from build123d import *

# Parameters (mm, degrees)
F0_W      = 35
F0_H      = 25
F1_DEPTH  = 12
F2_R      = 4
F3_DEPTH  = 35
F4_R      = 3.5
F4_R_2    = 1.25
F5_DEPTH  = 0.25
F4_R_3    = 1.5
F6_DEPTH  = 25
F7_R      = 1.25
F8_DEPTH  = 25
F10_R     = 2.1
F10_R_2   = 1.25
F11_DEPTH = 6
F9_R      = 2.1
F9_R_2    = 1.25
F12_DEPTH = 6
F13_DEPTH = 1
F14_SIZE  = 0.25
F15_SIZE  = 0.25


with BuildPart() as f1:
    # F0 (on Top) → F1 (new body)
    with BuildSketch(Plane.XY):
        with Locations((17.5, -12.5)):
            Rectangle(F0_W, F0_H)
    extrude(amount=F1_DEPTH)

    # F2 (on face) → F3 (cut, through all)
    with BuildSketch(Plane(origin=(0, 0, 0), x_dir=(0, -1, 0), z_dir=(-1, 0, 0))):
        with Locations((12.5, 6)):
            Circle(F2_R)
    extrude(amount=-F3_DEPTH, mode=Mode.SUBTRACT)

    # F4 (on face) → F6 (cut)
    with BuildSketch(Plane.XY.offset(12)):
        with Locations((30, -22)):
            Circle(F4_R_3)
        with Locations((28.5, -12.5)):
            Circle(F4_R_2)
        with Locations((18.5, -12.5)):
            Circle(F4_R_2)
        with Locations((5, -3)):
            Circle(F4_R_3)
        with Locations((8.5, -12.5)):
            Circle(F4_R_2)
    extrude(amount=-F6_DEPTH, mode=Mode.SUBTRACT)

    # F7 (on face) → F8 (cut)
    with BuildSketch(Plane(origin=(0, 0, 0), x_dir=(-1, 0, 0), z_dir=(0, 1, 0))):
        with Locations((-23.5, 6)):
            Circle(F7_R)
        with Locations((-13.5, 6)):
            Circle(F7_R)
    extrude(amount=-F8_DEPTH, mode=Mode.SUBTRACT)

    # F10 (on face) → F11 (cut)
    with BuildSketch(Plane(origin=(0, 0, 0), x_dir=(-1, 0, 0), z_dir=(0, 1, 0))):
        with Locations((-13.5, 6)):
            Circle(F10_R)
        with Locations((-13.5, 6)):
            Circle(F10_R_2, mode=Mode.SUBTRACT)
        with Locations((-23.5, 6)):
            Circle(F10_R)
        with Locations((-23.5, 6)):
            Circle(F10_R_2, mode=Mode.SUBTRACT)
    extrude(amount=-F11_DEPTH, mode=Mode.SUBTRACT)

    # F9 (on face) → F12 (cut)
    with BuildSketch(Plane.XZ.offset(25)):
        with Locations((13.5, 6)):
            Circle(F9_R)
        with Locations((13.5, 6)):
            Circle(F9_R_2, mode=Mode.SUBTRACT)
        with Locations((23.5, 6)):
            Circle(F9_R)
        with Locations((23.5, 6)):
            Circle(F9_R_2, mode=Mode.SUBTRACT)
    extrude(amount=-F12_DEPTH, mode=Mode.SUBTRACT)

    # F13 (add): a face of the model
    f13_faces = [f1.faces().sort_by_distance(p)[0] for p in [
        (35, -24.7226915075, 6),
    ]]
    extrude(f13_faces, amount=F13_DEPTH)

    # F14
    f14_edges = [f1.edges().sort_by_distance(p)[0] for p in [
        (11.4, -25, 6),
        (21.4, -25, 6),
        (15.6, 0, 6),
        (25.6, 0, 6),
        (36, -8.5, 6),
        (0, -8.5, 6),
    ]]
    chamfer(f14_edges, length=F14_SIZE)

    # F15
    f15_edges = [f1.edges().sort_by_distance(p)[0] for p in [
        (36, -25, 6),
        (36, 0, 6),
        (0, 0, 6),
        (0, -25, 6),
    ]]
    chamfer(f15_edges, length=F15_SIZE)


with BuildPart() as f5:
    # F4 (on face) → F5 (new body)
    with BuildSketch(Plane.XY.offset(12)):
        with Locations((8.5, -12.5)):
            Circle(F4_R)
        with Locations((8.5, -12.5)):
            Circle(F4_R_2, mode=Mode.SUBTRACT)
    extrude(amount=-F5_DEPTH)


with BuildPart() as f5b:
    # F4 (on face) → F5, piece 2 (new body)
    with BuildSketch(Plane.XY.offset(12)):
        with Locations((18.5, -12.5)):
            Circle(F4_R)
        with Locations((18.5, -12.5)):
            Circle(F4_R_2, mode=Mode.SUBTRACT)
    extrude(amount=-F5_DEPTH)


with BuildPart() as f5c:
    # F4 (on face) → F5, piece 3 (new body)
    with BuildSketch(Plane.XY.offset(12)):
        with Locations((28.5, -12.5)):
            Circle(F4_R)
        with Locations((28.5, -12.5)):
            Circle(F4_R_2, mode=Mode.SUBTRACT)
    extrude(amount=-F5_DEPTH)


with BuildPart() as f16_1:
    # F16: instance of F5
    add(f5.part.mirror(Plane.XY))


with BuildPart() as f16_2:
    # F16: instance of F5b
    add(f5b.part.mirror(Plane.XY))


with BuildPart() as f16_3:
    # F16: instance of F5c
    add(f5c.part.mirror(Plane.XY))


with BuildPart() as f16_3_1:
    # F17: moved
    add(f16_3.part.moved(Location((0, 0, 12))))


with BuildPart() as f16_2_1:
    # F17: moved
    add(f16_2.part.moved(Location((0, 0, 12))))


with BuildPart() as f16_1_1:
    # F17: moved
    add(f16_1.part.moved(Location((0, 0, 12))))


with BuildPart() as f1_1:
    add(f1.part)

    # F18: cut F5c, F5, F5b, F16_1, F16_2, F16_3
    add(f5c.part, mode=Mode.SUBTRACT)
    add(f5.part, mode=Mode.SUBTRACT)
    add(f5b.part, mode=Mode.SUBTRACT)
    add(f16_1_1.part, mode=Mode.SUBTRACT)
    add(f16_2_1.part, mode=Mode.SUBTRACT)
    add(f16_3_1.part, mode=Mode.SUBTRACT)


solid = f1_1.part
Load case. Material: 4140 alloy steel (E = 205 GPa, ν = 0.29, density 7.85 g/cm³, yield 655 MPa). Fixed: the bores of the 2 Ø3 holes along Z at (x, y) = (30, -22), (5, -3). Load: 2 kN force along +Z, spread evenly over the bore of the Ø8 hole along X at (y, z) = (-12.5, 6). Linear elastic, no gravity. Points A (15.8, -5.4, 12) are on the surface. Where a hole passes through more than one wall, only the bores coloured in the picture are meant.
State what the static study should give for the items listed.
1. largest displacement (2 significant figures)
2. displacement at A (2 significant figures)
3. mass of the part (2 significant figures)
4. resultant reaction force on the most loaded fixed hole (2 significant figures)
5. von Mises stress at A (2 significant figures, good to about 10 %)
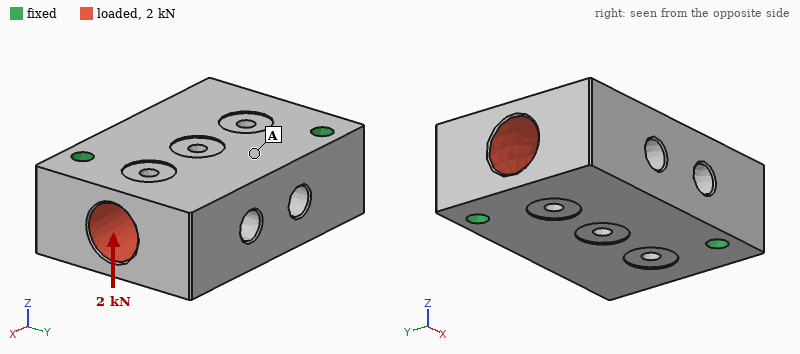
3.3 µm
1.6 µm
65 g
1.0 kN
5.9 MPa
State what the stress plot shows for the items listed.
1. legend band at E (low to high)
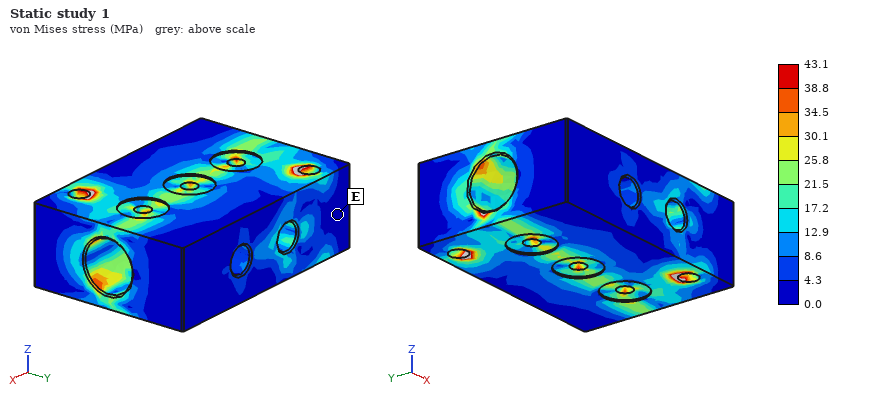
0.0 to 4.3 MPa
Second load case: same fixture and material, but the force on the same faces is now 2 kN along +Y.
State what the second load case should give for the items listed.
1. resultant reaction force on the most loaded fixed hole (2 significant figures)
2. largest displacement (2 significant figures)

1.0 kN
0.97 µm
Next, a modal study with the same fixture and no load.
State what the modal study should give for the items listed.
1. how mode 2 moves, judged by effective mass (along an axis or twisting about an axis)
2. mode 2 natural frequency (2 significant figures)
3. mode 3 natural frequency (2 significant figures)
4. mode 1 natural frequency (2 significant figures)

along Z
18 kHz
30 kHz
14 kHz
